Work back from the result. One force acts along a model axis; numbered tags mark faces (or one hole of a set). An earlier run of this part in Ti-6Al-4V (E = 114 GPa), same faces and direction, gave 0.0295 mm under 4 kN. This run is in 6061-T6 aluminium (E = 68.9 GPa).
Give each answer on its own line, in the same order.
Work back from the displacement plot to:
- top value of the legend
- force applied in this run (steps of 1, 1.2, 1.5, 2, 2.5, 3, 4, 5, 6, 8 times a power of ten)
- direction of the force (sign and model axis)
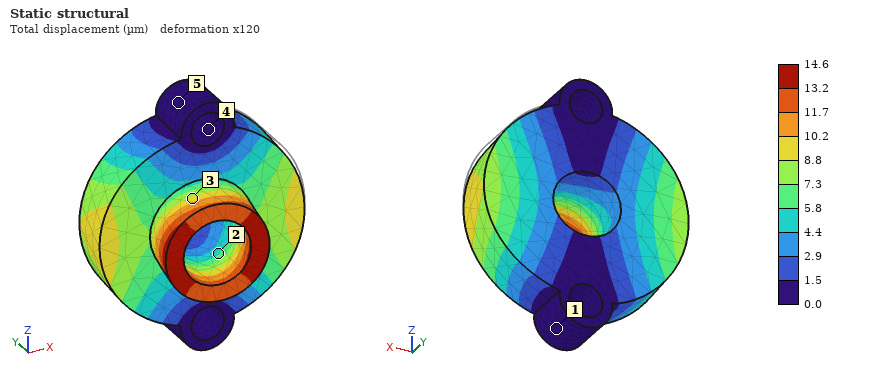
14.6 µm
1.2 kN
-X
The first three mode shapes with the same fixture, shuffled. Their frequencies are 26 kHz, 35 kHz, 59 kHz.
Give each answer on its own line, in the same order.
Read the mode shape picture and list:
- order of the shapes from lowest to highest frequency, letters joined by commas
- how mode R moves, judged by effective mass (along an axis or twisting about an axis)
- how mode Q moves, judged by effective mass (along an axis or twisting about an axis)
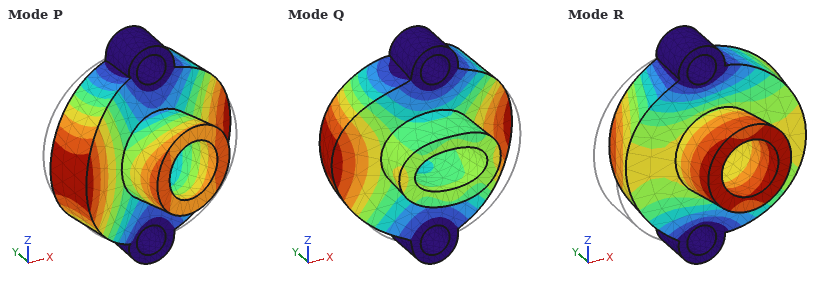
P, Q, R
along X
along Y
